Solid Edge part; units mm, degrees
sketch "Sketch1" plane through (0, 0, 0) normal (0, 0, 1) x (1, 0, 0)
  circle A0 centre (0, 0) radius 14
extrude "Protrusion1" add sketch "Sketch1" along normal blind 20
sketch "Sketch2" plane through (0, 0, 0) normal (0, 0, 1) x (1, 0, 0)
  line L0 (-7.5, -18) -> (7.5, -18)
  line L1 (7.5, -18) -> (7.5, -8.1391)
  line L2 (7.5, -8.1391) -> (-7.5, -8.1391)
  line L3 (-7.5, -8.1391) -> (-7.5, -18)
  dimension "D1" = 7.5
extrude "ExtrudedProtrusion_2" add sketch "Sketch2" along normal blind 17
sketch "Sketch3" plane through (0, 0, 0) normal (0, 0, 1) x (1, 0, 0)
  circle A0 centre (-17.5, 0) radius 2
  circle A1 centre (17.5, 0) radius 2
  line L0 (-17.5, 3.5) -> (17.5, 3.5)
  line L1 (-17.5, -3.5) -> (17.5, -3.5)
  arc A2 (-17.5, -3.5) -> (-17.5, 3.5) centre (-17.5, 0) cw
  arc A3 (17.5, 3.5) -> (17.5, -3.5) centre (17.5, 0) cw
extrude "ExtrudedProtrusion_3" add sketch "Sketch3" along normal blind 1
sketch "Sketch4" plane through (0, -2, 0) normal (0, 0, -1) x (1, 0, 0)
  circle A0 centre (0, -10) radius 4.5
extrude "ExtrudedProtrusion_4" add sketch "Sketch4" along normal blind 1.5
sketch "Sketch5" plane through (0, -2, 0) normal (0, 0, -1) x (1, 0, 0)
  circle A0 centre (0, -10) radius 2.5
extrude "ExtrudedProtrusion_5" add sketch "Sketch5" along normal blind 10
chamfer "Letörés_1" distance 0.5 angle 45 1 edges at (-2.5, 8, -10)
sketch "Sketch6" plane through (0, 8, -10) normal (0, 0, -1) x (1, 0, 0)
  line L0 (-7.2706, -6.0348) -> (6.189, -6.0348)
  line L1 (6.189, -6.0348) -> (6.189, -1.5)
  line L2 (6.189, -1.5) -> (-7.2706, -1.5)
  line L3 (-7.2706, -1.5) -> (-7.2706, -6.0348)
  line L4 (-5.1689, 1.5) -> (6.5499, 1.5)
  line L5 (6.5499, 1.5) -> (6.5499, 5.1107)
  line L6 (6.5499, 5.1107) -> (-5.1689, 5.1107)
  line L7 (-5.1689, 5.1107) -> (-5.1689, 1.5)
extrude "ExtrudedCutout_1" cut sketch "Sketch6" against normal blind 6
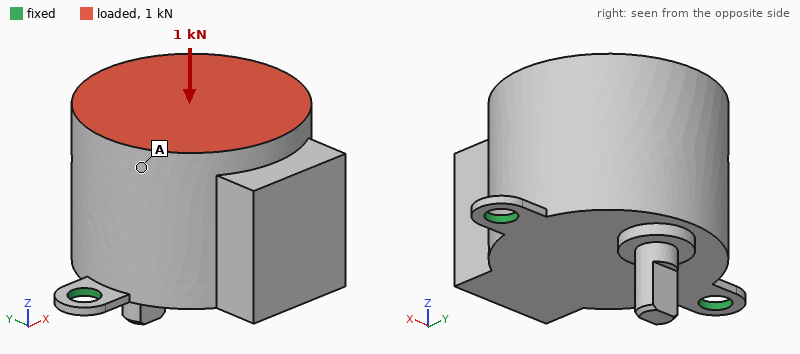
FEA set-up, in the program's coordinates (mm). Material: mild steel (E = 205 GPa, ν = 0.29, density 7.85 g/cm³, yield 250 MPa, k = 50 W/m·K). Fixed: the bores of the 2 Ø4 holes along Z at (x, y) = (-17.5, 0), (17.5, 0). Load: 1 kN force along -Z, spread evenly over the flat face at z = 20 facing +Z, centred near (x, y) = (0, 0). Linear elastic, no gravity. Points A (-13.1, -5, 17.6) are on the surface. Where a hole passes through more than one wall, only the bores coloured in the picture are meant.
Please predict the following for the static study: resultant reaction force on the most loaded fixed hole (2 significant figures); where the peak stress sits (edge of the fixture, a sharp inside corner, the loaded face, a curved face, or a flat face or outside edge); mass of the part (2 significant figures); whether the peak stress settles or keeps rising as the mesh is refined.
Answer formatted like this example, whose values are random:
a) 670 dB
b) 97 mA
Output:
a) 580 N
b) edge of the fixture
c) 110 g
d) keeps rising
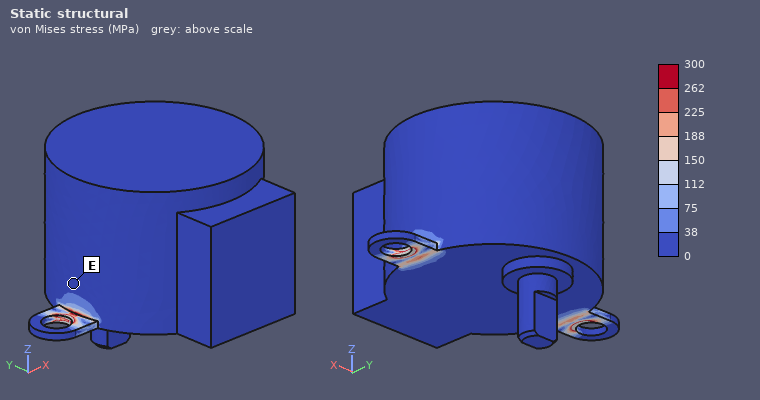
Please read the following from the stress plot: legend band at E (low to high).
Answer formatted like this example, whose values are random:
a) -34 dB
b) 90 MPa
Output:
a) 0 to 38 MPa
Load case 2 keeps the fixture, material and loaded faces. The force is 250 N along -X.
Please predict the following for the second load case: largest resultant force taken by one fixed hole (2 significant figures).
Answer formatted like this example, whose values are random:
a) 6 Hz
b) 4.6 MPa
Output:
a) 210 N
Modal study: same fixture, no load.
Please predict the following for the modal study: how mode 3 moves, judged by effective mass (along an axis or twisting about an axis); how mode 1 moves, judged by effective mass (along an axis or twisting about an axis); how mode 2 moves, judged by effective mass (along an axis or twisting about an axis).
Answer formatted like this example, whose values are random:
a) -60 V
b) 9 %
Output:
a) along X
b) along Y
c) along Z
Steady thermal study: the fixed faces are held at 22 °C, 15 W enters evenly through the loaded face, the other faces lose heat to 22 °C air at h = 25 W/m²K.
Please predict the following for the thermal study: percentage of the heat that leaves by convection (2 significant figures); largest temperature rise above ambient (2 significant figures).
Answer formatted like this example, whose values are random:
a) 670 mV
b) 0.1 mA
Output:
a) 28 %
b) 64 K
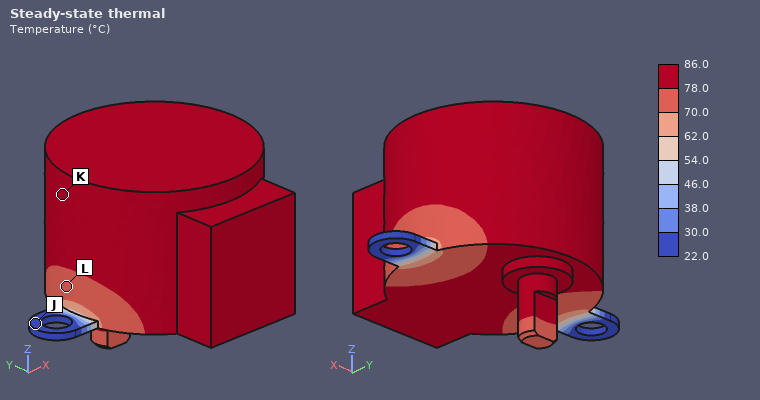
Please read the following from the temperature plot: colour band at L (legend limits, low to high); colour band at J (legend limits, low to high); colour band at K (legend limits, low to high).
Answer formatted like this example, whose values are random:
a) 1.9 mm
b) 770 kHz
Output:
a) 70.0 to 78.0 °C
b) 22.0 to 30.0 °C
c) 78.0 to 86.0 °C
